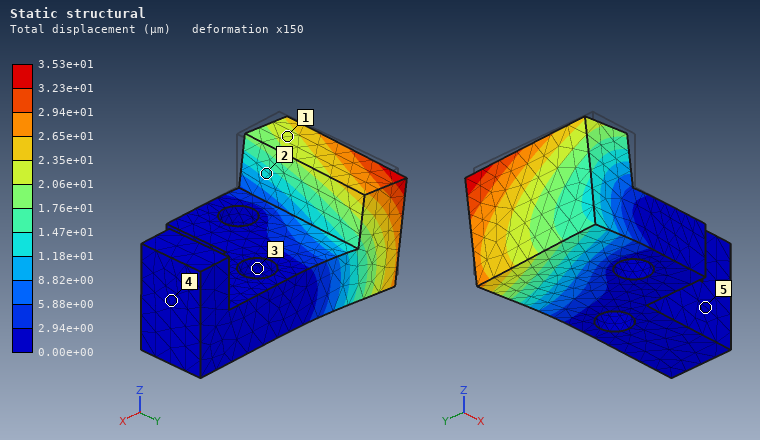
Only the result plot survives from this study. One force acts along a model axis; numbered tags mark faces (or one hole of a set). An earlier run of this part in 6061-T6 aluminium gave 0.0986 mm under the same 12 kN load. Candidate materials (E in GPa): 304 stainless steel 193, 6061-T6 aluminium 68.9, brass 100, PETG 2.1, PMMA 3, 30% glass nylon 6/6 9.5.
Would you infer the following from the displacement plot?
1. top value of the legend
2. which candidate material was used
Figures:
3.53e+01 µm
304 stainless steel
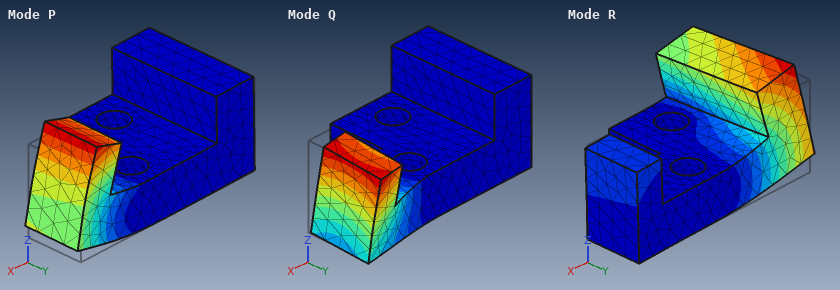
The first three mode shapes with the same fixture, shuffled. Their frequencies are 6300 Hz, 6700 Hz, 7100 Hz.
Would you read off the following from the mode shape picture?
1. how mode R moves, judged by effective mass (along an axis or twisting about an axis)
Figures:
along Z
